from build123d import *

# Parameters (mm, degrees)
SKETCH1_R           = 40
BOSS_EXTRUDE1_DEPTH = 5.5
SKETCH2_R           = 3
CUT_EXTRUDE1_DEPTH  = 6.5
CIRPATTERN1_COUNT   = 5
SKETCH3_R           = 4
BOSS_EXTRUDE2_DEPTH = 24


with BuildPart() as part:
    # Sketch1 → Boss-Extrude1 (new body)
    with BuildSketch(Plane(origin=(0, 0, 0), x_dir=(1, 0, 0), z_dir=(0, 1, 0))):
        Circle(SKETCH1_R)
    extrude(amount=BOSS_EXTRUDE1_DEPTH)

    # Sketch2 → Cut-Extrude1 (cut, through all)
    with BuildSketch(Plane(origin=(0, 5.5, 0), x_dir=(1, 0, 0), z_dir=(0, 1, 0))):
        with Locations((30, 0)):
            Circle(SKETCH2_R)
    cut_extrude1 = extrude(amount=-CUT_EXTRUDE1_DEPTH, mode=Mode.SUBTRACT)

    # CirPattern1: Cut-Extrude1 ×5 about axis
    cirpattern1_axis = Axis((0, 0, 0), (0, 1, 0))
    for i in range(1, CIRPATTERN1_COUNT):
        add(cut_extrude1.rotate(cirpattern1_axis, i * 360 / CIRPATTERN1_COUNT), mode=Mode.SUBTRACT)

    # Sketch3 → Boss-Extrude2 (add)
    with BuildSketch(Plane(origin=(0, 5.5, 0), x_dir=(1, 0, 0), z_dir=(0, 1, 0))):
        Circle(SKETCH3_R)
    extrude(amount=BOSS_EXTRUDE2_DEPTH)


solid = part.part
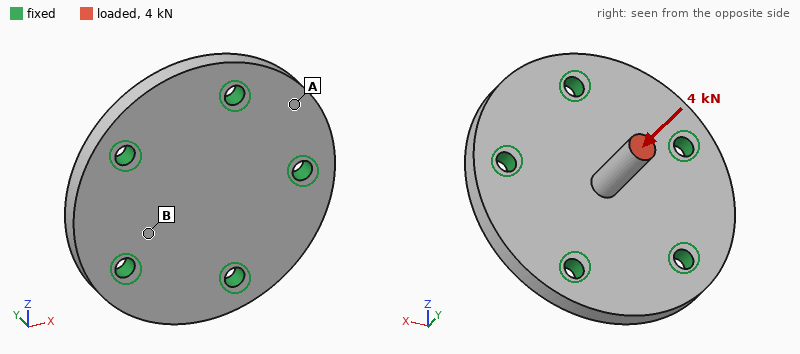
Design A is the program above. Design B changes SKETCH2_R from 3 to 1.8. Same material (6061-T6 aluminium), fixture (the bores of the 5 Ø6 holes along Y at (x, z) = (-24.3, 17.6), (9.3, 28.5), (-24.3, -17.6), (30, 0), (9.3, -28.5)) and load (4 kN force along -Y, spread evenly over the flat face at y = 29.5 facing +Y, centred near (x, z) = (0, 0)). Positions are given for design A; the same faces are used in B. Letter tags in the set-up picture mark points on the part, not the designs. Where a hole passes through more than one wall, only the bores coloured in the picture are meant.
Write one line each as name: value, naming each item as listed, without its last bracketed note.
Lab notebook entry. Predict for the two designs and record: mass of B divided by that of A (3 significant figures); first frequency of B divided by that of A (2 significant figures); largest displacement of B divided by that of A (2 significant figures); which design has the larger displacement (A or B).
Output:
mass of B divided by that of A: 1.02
first frequency of B divided by that of A: 1.0
largest displacement of B divided by that of A: 1.1
which design has the larger displacement: B
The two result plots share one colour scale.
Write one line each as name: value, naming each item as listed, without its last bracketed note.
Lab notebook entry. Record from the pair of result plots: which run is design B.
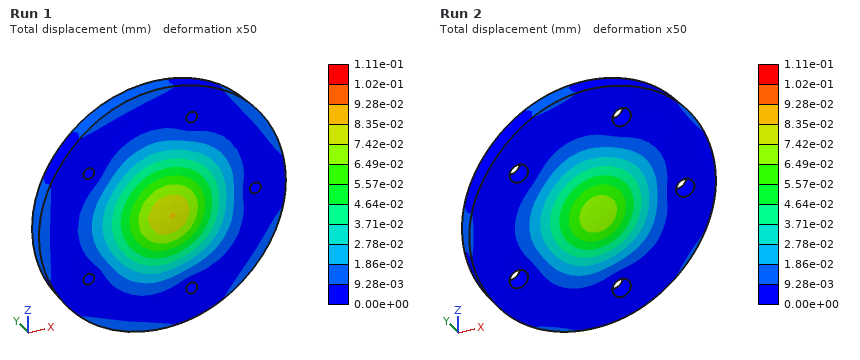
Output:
which run is design B: Run 1
